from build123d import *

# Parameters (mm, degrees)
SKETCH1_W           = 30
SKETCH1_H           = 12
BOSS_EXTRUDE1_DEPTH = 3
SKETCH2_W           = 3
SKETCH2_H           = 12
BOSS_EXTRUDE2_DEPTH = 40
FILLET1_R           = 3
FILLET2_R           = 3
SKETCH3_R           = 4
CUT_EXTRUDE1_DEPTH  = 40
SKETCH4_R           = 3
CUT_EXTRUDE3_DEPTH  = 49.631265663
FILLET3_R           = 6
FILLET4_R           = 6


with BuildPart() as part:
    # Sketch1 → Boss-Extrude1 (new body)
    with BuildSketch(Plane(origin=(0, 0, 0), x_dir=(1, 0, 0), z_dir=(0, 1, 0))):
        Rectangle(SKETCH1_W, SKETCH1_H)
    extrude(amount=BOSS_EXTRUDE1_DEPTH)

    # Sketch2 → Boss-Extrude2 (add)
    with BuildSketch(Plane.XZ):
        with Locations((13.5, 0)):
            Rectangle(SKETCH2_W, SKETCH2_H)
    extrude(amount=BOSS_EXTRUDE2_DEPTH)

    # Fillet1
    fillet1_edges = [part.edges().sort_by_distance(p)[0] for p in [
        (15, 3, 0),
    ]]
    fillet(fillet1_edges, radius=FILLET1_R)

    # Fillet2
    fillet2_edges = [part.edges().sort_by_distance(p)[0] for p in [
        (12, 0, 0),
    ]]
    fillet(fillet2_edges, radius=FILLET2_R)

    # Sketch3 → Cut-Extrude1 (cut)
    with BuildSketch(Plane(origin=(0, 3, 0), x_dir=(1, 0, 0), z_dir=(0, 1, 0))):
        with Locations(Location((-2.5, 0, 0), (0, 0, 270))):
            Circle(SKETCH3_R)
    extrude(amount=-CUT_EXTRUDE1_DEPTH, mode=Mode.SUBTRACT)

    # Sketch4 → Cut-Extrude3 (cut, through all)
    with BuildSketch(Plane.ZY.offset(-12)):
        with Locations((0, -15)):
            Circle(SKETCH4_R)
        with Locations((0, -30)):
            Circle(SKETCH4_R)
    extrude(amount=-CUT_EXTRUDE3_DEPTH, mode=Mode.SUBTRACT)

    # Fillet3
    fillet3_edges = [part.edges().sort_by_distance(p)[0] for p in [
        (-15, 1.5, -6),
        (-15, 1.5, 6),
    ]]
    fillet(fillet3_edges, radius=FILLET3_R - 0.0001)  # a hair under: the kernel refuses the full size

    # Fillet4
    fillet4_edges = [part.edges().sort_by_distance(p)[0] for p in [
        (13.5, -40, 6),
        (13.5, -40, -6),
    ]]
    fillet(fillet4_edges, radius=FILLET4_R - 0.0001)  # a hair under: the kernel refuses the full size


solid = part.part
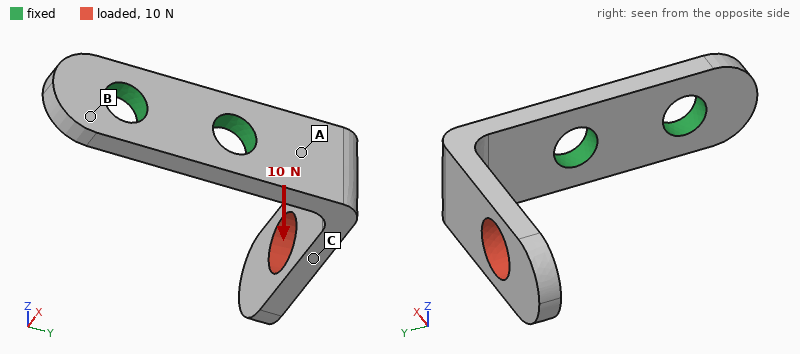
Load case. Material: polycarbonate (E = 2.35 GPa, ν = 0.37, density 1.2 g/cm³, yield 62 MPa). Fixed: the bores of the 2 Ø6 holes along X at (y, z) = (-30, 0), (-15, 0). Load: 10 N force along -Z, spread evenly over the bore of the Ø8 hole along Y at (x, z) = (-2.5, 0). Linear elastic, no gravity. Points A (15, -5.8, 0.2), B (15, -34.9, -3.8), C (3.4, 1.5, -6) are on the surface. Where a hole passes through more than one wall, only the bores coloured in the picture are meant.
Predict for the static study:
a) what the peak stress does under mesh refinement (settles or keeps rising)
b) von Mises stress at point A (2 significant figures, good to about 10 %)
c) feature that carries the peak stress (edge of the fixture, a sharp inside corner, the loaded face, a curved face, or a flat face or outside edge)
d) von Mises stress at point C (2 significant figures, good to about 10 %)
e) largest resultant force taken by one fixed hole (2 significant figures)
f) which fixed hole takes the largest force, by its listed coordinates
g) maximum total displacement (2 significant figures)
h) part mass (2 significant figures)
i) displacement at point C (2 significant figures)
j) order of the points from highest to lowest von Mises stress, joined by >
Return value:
keeps rising
6.5 MPa
edge of the fixture
1.5 MPa
12 N
(-15, 0)
0.64 mm
2.5 g
0.26 mm
A > C > B
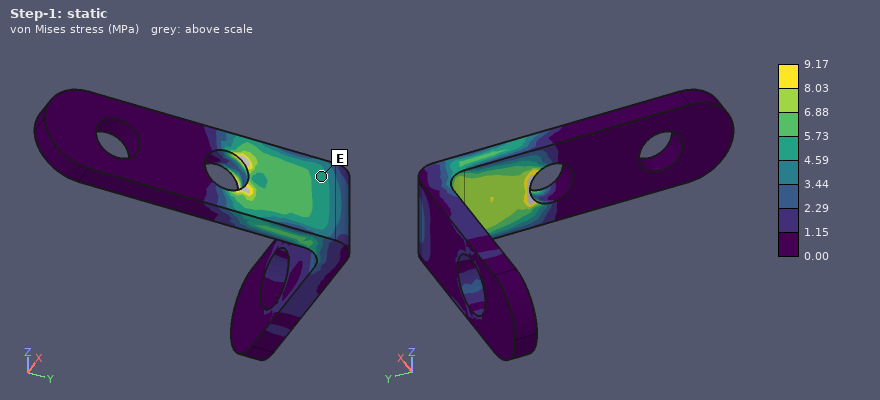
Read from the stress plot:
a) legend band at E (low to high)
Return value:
4.59 to 5.73 MPa
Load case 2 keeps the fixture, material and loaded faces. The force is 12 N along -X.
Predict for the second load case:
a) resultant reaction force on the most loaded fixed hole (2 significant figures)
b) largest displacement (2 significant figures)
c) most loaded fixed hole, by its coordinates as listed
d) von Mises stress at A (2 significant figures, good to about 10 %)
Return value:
12 N
0.56 mm
(-15, 0)
4.4 MPa
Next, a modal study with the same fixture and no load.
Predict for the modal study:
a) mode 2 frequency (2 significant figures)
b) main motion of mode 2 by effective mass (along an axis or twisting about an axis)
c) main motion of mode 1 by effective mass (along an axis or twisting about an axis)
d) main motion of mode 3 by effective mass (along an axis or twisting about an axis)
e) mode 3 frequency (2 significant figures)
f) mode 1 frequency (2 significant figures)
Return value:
830 Hz
along Z
along Y
along X
1800 Hz
560 Hz
